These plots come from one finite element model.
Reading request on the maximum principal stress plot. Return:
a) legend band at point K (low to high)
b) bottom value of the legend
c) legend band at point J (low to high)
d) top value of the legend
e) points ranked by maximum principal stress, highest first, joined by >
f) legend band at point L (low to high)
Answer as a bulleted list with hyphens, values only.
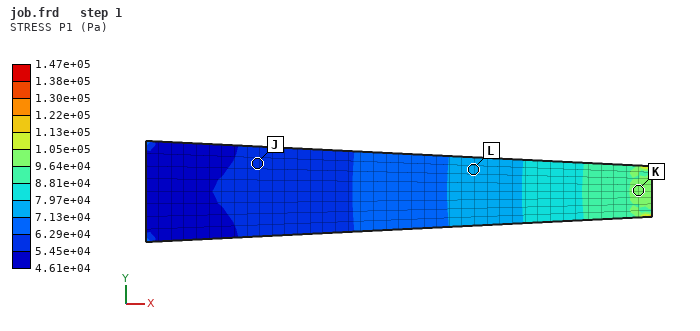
- 9.64e+04 to 1.05e+05 Pa
- 4.61e+04 Pa
- 5.45e+04 to 6.29e+04 Pa
- 1.47e+05 Pa
- K > L > J
- 7.13e+04 to 7.97e+04 Pa
